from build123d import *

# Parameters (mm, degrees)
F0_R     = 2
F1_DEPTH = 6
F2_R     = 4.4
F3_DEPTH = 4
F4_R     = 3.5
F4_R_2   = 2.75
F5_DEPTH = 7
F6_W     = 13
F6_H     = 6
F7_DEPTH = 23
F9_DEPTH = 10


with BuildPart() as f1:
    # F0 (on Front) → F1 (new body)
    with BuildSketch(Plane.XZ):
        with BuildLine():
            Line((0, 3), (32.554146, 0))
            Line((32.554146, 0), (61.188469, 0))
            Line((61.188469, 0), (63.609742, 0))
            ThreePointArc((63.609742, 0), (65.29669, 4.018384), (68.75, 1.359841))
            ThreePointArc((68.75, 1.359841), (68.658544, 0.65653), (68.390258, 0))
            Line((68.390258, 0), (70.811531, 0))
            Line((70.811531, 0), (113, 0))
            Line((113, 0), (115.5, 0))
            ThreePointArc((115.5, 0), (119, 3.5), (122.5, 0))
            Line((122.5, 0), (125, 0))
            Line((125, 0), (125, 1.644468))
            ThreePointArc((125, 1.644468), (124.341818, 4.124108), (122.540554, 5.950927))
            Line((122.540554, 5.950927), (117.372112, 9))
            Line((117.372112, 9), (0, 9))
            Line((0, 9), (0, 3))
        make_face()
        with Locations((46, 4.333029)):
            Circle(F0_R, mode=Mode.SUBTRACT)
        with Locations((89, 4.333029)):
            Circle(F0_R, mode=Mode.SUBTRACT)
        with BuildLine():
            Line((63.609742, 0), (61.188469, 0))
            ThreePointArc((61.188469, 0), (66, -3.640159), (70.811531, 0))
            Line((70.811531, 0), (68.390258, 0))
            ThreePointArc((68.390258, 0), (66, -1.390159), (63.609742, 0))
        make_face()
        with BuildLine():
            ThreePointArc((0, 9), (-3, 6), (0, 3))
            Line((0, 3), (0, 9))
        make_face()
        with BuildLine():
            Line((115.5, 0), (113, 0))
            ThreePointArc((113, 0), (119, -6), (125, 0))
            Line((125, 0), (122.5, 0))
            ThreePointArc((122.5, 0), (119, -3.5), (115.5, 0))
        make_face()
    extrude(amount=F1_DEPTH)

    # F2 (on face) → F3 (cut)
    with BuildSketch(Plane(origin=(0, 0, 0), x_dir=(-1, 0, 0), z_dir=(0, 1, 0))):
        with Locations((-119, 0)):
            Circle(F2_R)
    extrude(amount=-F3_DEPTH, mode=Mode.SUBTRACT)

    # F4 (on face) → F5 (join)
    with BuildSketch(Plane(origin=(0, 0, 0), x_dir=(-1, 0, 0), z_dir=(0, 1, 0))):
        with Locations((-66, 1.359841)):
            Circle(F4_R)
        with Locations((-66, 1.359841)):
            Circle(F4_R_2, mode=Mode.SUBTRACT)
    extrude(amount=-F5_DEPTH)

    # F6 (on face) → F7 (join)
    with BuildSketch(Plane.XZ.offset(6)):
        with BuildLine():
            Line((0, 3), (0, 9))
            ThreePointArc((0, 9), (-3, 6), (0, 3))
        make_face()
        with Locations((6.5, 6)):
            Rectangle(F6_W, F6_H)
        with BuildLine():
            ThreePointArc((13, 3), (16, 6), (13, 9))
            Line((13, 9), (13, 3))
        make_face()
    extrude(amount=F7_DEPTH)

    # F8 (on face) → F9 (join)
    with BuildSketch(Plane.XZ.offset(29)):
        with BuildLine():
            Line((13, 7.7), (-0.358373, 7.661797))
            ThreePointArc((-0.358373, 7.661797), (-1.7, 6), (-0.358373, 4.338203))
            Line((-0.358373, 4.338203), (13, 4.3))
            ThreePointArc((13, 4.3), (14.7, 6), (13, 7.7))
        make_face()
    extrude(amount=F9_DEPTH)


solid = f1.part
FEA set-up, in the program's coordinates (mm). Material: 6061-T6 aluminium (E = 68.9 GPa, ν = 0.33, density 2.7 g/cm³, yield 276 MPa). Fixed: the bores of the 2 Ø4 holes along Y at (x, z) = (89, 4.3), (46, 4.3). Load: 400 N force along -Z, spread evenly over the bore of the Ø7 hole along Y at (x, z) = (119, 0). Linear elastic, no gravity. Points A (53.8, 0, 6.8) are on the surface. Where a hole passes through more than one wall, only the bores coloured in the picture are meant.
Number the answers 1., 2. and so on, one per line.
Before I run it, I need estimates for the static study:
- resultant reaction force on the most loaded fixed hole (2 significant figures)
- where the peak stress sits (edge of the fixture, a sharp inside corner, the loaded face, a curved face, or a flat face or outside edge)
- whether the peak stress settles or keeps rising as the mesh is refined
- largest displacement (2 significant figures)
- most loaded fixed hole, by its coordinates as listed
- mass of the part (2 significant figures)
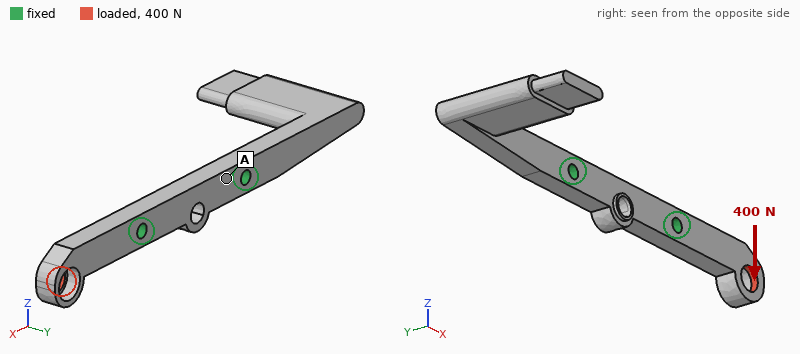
1. 450 N
2. edge of the fixture
3. keeps rising
4. 0.24 mm
5. (89, 4.3)
6. 25 g
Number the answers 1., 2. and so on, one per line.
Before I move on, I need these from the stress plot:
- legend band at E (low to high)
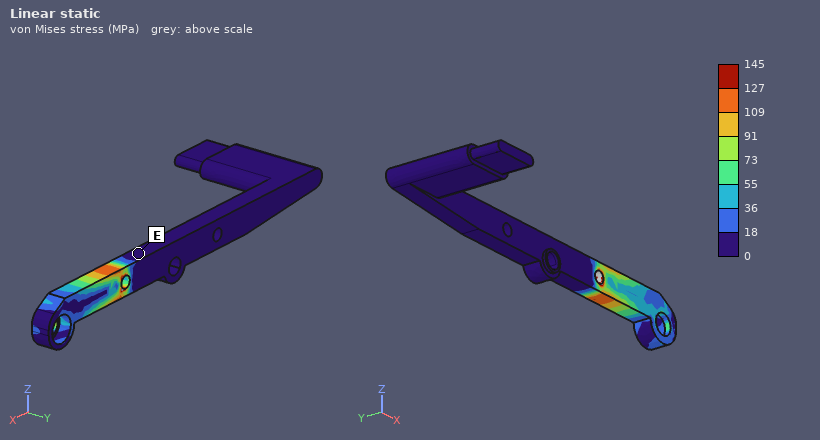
1. 0 to 18 MPa
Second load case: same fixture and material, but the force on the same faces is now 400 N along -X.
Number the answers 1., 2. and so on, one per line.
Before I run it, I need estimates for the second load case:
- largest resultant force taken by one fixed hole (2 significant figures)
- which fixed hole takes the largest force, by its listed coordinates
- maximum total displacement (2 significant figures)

1. 400 N
2. (89, 4.3)
3. 76 µm
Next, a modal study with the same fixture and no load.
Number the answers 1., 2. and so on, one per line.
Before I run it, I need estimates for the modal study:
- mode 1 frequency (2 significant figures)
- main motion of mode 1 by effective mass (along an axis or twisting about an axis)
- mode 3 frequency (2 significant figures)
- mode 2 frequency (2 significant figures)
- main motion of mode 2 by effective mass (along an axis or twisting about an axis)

1. 960 Hz
2. along Y
3. 3000 Hz
4. 1100 Hz
5. along Z
